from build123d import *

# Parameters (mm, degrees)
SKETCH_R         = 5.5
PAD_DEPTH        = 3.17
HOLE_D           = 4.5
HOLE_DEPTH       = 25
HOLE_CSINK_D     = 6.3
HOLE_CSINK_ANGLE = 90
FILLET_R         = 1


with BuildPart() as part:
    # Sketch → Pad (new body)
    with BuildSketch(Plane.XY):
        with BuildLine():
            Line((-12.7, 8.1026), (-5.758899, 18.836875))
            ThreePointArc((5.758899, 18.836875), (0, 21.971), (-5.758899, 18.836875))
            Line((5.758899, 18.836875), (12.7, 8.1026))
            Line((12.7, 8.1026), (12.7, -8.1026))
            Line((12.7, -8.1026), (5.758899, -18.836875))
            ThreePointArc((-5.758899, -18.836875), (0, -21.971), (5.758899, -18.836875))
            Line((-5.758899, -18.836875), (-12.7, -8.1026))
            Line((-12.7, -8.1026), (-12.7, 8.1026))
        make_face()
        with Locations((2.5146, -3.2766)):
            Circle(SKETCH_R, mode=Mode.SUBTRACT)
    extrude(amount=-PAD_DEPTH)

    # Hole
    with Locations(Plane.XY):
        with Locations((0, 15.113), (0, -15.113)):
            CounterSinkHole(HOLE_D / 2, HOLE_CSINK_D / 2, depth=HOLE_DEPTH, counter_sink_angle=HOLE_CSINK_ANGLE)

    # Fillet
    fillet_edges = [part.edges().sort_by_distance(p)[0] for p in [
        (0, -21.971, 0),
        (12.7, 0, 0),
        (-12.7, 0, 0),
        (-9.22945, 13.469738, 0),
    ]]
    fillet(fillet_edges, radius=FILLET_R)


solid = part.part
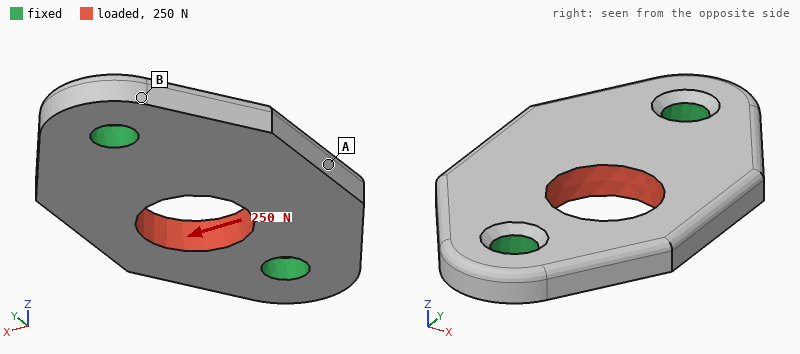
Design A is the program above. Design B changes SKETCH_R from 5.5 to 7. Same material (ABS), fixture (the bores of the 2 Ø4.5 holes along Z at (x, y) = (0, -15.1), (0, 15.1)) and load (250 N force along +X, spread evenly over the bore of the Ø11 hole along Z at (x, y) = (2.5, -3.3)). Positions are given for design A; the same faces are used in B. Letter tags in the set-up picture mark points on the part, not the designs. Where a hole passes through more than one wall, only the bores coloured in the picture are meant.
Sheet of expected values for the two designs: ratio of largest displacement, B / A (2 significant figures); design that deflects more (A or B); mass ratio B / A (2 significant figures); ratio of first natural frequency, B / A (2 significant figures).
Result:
1.2
B
0.92
1.0
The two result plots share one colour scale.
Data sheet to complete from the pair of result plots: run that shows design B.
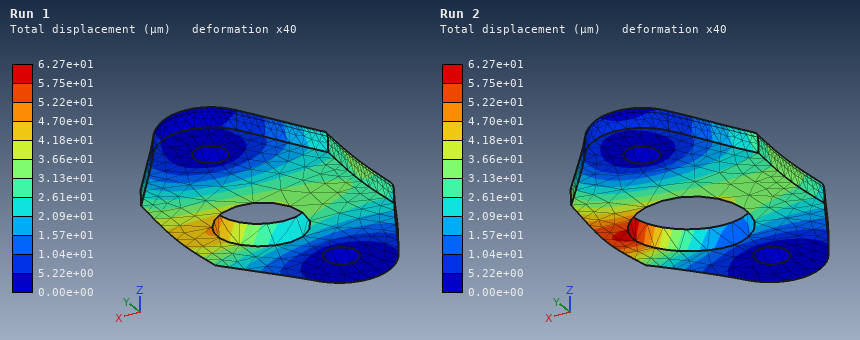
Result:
Run 2
